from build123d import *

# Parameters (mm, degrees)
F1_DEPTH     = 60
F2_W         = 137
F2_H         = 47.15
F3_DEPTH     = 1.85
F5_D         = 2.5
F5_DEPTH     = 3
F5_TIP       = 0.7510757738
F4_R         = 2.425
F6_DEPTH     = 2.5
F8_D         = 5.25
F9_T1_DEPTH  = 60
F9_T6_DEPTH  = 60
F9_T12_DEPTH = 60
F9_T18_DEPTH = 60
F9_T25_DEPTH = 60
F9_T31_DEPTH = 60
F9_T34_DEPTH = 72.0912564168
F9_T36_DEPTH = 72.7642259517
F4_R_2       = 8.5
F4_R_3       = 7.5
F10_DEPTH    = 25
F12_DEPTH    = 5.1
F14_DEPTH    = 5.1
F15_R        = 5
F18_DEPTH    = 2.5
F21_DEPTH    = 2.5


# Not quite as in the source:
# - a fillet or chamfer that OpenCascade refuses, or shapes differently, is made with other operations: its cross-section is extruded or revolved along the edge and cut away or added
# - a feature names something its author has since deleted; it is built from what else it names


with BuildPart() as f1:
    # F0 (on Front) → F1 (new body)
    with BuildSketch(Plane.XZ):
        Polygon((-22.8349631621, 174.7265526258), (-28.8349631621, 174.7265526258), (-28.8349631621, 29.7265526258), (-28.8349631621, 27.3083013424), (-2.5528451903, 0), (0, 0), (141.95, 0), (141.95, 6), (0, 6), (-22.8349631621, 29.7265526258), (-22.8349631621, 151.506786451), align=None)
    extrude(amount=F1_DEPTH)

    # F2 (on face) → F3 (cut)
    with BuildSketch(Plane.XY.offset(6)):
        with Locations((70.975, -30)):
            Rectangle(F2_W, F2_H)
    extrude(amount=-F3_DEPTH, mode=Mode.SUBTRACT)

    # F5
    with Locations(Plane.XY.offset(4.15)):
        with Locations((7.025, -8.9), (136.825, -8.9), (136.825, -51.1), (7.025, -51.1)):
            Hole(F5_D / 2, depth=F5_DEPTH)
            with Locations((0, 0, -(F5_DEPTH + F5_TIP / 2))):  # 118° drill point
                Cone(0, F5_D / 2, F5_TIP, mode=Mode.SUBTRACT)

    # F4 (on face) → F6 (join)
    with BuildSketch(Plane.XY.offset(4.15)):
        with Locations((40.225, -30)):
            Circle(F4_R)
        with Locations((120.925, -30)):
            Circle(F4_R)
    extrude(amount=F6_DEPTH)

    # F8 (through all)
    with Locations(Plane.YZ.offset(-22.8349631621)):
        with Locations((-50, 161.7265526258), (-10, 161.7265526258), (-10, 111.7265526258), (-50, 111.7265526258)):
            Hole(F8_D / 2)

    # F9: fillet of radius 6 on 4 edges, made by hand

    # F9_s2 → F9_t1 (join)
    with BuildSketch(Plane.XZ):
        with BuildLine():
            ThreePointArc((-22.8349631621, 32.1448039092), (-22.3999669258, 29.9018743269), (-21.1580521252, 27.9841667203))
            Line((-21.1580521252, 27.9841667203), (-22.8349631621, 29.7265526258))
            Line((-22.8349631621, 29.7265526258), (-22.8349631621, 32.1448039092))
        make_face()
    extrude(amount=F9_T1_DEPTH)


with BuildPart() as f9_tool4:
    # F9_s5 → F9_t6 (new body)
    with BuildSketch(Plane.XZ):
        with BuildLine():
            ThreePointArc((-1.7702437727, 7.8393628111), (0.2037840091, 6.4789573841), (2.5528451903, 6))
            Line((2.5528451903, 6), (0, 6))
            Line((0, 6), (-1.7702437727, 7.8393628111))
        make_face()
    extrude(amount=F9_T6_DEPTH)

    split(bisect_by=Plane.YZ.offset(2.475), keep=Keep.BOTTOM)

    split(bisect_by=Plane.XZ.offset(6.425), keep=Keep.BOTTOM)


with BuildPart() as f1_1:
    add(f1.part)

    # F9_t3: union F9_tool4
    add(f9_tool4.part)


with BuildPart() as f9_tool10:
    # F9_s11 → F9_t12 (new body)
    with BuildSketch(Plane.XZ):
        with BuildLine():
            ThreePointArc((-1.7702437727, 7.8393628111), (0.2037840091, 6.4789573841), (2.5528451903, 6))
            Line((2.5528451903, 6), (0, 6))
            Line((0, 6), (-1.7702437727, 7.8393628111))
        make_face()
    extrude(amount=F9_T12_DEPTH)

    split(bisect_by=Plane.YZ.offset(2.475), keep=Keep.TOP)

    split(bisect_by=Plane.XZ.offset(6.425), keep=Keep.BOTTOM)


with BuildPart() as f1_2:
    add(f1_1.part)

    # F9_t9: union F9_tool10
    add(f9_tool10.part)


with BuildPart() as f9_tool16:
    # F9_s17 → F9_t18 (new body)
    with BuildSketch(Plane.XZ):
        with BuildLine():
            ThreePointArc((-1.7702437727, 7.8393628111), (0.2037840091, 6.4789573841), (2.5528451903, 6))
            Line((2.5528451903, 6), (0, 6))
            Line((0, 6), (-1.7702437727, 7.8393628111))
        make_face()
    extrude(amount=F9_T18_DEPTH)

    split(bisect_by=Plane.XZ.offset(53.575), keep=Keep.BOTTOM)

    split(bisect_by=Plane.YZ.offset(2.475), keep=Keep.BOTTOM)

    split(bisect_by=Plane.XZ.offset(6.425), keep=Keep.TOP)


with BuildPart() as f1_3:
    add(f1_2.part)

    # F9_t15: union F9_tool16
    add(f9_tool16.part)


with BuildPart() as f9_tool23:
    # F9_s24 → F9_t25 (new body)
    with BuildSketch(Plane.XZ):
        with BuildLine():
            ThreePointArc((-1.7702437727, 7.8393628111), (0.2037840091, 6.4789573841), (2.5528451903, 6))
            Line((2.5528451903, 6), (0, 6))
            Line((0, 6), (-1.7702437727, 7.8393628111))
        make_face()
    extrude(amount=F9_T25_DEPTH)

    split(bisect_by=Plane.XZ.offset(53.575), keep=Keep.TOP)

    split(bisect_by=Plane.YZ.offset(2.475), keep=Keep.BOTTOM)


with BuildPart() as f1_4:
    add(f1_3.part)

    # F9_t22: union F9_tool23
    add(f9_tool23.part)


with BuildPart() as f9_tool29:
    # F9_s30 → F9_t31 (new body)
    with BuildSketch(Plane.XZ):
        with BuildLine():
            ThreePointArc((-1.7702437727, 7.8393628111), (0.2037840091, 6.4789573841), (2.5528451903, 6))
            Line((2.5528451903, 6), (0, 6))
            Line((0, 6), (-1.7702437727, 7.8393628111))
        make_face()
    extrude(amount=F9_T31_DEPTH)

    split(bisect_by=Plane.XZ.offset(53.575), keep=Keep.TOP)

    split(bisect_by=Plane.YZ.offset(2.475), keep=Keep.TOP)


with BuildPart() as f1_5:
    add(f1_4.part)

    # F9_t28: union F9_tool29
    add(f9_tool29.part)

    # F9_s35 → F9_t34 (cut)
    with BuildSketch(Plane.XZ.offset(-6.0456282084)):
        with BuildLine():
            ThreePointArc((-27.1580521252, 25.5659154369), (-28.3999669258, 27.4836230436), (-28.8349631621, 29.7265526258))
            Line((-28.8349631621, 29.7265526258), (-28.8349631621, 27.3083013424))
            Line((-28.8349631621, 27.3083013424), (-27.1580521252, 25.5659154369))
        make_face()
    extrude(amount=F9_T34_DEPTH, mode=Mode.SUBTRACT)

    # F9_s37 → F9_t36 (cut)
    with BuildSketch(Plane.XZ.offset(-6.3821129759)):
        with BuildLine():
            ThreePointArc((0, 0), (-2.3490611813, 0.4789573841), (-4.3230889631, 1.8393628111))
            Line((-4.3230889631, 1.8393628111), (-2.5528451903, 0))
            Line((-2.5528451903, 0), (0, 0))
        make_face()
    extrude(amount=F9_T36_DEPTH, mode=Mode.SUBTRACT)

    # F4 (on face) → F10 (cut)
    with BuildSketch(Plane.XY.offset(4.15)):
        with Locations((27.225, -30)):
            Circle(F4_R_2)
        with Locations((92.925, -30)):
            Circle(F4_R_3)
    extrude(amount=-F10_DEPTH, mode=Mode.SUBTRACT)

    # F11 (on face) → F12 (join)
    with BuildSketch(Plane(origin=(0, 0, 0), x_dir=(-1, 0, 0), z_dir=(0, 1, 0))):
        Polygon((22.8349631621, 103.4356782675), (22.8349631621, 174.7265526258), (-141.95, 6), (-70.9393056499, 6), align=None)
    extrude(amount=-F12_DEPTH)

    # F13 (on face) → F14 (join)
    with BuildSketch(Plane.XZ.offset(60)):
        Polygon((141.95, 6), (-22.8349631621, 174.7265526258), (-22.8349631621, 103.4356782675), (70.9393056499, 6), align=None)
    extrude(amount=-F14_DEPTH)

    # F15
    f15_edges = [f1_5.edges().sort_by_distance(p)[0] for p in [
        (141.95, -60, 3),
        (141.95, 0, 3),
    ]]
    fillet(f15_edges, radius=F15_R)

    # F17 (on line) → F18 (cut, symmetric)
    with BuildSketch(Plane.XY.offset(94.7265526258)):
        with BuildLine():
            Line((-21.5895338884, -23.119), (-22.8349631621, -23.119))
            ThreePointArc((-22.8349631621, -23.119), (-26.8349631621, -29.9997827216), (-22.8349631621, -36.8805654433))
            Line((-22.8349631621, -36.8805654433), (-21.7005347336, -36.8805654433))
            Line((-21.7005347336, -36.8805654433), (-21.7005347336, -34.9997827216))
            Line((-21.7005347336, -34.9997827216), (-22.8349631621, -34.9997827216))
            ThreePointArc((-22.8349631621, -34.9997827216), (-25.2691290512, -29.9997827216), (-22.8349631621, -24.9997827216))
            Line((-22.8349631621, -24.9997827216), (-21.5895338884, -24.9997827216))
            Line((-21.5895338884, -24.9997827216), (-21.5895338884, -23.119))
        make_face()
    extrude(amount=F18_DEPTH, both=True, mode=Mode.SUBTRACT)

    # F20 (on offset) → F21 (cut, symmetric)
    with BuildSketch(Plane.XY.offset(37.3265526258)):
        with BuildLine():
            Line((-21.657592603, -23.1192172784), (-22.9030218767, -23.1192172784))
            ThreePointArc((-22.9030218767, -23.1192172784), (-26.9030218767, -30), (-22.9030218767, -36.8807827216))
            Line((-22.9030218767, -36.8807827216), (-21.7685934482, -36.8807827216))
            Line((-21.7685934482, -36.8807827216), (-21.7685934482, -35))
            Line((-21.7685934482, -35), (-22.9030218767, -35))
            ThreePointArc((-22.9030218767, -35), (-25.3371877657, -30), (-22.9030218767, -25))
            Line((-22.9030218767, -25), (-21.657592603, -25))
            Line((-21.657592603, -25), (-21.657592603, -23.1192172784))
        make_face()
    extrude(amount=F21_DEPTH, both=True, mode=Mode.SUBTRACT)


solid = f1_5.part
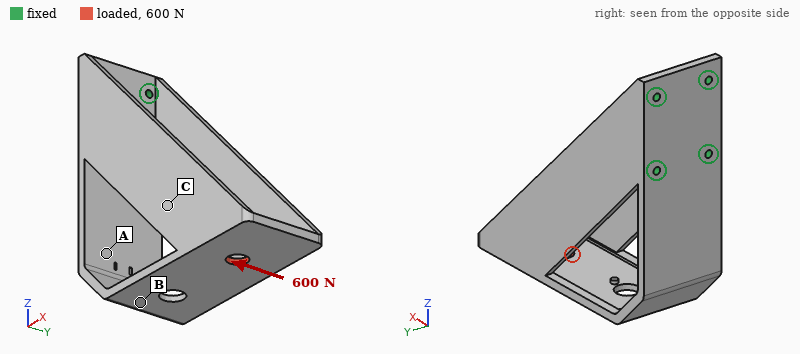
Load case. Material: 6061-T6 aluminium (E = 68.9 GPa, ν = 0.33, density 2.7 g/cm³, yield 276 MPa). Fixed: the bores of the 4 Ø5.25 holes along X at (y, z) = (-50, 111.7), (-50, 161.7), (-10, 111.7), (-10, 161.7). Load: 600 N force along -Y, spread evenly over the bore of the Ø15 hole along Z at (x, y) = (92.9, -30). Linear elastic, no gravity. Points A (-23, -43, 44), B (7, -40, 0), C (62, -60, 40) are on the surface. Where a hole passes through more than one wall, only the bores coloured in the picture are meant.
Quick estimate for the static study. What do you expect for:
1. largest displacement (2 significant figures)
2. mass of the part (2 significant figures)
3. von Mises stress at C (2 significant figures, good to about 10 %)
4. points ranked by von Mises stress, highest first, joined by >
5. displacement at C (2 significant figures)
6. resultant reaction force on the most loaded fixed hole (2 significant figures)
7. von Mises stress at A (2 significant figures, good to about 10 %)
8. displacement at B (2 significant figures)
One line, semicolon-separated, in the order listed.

1.5 mm; 530 g; 14 MPa; A > C > B; 0.80 mm; 3.0 kN; 27 MPa; 0.30 mm
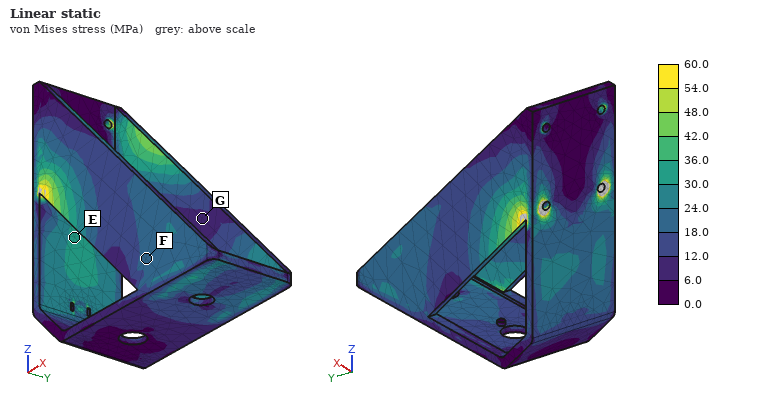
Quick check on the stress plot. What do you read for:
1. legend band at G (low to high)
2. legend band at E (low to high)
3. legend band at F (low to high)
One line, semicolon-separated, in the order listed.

6.0 to 12.0 MPa; 30.0 to 36.0 MPa; 18.0 to 24.0 MPa
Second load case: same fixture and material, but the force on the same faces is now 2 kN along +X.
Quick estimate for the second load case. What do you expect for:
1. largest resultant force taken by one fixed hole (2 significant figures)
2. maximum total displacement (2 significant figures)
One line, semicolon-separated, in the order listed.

3.2 kN; 0.59 mm
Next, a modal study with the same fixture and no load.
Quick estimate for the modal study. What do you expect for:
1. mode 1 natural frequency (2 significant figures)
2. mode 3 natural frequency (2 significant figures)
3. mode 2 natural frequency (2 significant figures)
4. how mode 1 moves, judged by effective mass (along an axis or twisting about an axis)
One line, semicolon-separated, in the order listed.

260 Hz; 740 Hz; 660 Hz; along Y
